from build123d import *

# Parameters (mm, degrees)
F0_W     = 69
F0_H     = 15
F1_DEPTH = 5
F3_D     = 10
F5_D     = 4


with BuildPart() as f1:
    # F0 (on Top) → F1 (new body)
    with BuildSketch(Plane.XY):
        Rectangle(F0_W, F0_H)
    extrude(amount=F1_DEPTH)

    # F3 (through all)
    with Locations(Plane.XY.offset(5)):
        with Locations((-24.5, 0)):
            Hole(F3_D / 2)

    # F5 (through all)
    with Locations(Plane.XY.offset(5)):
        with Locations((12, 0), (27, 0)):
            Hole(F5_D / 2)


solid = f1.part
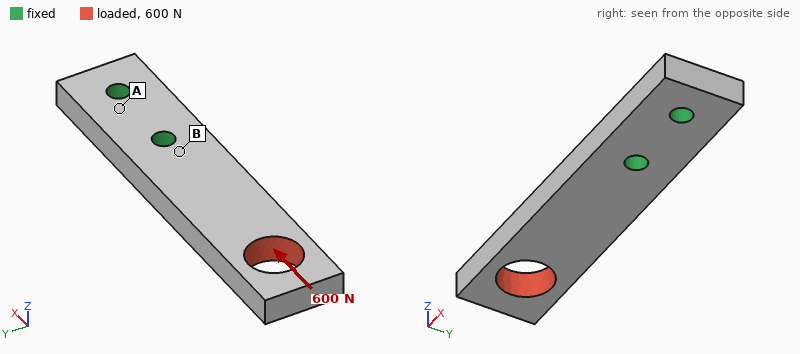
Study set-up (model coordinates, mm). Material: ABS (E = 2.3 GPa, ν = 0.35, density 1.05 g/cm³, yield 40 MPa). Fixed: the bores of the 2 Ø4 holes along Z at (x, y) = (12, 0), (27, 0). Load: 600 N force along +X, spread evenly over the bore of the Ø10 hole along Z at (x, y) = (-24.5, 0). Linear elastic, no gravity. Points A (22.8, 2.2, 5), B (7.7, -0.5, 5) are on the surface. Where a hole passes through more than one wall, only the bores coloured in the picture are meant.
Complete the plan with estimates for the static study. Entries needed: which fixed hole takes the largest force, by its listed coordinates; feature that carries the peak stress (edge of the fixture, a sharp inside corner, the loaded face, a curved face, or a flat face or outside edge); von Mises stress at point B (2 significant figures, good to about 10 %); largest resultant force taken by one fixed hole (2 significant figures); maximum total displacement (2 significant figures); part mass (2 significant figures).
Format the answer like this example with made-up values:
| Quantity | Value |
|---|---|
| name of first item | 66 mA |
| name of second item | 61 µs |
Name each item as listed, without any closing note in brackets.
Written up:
| Quantity | Value |
|---|---|
| which fixed hole takes the largest force, by its listed coordinates | (12, 0) |
| feature that carries the peak stress | the loaded face |
| von Mises stress at point B | 12 MPa |
| largest resultant force taken by one fixed hole | 520 N |
| maximum total displacement | 0.22 mm |
| part mass | 4.9 g |
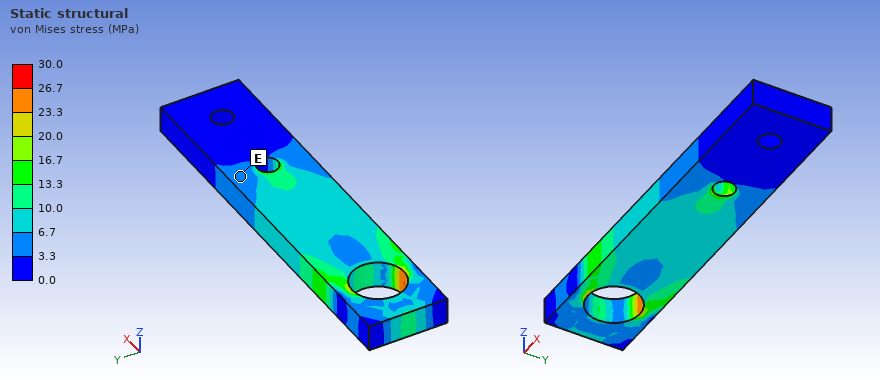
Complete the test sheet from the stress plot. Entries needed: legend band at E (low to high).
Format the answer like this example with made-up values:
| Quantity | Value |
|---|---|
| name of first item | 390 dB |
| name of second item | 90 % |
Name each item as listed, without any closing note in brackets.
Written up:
| Quantity | Value |
|---|---|
| legend band at E | 3.3 to 6.7 MPa |
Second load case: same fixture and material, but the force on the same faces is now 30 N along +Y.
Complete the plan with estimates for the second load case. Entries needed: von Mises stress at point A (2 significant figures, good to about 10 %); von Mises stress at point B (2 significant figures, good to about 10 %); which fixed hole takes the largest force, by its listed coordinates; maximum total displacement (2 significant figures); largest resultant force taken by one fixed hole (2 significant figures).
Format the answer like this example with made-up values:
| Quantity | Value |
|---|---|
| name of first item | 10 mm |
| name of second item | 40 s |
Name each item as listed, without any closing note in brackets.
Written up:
| Quantity | Value |
|---|---|
| von Mises stress at point A | 1.4 MPa |
| von Mises stress at point B | 1.9 MPa |
| which fixed hole takes the largest force, by its listed coordinates | (12, 0) |
| maximum total displacement | 0.35 mm |
| largest resultant force taken by one fixed hole | 72 N |
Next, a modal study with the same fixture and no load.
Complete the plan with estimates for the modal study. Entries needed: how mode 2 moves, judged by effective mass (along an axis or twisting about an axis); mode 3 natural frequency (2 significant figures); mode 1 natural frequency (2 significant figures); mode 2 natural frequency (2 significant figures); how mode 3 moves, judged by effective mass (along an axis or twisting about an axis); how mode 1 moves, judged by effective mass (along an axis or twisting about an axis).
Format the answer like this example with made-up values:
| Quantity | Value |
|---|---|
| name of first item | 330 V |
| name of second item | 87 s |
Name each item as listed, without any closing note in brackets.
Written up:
| Quantity | Value |
|---|---|
| how mode 2 moves, judged by effective mass | along Y |
| mode 3 natural frequency | 2800 Hz |
| mode 1 natural frequency | 630 Hz |
| mode 2 natural frequency | 1400 Hz |
| how mode 3 moves, judged by effective mass | twisting about X |
| how mode 1 moves, judged by effective mass | along Z |
